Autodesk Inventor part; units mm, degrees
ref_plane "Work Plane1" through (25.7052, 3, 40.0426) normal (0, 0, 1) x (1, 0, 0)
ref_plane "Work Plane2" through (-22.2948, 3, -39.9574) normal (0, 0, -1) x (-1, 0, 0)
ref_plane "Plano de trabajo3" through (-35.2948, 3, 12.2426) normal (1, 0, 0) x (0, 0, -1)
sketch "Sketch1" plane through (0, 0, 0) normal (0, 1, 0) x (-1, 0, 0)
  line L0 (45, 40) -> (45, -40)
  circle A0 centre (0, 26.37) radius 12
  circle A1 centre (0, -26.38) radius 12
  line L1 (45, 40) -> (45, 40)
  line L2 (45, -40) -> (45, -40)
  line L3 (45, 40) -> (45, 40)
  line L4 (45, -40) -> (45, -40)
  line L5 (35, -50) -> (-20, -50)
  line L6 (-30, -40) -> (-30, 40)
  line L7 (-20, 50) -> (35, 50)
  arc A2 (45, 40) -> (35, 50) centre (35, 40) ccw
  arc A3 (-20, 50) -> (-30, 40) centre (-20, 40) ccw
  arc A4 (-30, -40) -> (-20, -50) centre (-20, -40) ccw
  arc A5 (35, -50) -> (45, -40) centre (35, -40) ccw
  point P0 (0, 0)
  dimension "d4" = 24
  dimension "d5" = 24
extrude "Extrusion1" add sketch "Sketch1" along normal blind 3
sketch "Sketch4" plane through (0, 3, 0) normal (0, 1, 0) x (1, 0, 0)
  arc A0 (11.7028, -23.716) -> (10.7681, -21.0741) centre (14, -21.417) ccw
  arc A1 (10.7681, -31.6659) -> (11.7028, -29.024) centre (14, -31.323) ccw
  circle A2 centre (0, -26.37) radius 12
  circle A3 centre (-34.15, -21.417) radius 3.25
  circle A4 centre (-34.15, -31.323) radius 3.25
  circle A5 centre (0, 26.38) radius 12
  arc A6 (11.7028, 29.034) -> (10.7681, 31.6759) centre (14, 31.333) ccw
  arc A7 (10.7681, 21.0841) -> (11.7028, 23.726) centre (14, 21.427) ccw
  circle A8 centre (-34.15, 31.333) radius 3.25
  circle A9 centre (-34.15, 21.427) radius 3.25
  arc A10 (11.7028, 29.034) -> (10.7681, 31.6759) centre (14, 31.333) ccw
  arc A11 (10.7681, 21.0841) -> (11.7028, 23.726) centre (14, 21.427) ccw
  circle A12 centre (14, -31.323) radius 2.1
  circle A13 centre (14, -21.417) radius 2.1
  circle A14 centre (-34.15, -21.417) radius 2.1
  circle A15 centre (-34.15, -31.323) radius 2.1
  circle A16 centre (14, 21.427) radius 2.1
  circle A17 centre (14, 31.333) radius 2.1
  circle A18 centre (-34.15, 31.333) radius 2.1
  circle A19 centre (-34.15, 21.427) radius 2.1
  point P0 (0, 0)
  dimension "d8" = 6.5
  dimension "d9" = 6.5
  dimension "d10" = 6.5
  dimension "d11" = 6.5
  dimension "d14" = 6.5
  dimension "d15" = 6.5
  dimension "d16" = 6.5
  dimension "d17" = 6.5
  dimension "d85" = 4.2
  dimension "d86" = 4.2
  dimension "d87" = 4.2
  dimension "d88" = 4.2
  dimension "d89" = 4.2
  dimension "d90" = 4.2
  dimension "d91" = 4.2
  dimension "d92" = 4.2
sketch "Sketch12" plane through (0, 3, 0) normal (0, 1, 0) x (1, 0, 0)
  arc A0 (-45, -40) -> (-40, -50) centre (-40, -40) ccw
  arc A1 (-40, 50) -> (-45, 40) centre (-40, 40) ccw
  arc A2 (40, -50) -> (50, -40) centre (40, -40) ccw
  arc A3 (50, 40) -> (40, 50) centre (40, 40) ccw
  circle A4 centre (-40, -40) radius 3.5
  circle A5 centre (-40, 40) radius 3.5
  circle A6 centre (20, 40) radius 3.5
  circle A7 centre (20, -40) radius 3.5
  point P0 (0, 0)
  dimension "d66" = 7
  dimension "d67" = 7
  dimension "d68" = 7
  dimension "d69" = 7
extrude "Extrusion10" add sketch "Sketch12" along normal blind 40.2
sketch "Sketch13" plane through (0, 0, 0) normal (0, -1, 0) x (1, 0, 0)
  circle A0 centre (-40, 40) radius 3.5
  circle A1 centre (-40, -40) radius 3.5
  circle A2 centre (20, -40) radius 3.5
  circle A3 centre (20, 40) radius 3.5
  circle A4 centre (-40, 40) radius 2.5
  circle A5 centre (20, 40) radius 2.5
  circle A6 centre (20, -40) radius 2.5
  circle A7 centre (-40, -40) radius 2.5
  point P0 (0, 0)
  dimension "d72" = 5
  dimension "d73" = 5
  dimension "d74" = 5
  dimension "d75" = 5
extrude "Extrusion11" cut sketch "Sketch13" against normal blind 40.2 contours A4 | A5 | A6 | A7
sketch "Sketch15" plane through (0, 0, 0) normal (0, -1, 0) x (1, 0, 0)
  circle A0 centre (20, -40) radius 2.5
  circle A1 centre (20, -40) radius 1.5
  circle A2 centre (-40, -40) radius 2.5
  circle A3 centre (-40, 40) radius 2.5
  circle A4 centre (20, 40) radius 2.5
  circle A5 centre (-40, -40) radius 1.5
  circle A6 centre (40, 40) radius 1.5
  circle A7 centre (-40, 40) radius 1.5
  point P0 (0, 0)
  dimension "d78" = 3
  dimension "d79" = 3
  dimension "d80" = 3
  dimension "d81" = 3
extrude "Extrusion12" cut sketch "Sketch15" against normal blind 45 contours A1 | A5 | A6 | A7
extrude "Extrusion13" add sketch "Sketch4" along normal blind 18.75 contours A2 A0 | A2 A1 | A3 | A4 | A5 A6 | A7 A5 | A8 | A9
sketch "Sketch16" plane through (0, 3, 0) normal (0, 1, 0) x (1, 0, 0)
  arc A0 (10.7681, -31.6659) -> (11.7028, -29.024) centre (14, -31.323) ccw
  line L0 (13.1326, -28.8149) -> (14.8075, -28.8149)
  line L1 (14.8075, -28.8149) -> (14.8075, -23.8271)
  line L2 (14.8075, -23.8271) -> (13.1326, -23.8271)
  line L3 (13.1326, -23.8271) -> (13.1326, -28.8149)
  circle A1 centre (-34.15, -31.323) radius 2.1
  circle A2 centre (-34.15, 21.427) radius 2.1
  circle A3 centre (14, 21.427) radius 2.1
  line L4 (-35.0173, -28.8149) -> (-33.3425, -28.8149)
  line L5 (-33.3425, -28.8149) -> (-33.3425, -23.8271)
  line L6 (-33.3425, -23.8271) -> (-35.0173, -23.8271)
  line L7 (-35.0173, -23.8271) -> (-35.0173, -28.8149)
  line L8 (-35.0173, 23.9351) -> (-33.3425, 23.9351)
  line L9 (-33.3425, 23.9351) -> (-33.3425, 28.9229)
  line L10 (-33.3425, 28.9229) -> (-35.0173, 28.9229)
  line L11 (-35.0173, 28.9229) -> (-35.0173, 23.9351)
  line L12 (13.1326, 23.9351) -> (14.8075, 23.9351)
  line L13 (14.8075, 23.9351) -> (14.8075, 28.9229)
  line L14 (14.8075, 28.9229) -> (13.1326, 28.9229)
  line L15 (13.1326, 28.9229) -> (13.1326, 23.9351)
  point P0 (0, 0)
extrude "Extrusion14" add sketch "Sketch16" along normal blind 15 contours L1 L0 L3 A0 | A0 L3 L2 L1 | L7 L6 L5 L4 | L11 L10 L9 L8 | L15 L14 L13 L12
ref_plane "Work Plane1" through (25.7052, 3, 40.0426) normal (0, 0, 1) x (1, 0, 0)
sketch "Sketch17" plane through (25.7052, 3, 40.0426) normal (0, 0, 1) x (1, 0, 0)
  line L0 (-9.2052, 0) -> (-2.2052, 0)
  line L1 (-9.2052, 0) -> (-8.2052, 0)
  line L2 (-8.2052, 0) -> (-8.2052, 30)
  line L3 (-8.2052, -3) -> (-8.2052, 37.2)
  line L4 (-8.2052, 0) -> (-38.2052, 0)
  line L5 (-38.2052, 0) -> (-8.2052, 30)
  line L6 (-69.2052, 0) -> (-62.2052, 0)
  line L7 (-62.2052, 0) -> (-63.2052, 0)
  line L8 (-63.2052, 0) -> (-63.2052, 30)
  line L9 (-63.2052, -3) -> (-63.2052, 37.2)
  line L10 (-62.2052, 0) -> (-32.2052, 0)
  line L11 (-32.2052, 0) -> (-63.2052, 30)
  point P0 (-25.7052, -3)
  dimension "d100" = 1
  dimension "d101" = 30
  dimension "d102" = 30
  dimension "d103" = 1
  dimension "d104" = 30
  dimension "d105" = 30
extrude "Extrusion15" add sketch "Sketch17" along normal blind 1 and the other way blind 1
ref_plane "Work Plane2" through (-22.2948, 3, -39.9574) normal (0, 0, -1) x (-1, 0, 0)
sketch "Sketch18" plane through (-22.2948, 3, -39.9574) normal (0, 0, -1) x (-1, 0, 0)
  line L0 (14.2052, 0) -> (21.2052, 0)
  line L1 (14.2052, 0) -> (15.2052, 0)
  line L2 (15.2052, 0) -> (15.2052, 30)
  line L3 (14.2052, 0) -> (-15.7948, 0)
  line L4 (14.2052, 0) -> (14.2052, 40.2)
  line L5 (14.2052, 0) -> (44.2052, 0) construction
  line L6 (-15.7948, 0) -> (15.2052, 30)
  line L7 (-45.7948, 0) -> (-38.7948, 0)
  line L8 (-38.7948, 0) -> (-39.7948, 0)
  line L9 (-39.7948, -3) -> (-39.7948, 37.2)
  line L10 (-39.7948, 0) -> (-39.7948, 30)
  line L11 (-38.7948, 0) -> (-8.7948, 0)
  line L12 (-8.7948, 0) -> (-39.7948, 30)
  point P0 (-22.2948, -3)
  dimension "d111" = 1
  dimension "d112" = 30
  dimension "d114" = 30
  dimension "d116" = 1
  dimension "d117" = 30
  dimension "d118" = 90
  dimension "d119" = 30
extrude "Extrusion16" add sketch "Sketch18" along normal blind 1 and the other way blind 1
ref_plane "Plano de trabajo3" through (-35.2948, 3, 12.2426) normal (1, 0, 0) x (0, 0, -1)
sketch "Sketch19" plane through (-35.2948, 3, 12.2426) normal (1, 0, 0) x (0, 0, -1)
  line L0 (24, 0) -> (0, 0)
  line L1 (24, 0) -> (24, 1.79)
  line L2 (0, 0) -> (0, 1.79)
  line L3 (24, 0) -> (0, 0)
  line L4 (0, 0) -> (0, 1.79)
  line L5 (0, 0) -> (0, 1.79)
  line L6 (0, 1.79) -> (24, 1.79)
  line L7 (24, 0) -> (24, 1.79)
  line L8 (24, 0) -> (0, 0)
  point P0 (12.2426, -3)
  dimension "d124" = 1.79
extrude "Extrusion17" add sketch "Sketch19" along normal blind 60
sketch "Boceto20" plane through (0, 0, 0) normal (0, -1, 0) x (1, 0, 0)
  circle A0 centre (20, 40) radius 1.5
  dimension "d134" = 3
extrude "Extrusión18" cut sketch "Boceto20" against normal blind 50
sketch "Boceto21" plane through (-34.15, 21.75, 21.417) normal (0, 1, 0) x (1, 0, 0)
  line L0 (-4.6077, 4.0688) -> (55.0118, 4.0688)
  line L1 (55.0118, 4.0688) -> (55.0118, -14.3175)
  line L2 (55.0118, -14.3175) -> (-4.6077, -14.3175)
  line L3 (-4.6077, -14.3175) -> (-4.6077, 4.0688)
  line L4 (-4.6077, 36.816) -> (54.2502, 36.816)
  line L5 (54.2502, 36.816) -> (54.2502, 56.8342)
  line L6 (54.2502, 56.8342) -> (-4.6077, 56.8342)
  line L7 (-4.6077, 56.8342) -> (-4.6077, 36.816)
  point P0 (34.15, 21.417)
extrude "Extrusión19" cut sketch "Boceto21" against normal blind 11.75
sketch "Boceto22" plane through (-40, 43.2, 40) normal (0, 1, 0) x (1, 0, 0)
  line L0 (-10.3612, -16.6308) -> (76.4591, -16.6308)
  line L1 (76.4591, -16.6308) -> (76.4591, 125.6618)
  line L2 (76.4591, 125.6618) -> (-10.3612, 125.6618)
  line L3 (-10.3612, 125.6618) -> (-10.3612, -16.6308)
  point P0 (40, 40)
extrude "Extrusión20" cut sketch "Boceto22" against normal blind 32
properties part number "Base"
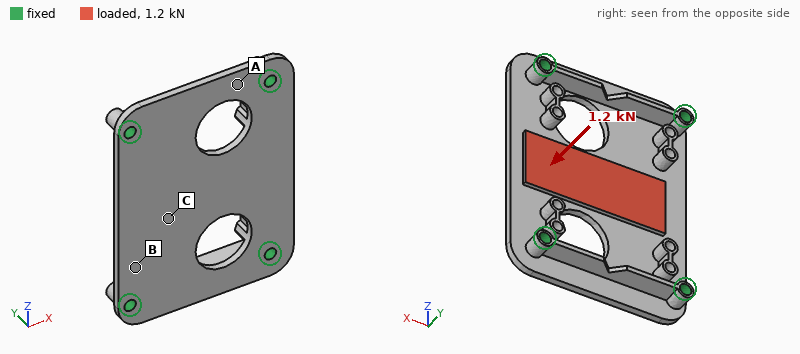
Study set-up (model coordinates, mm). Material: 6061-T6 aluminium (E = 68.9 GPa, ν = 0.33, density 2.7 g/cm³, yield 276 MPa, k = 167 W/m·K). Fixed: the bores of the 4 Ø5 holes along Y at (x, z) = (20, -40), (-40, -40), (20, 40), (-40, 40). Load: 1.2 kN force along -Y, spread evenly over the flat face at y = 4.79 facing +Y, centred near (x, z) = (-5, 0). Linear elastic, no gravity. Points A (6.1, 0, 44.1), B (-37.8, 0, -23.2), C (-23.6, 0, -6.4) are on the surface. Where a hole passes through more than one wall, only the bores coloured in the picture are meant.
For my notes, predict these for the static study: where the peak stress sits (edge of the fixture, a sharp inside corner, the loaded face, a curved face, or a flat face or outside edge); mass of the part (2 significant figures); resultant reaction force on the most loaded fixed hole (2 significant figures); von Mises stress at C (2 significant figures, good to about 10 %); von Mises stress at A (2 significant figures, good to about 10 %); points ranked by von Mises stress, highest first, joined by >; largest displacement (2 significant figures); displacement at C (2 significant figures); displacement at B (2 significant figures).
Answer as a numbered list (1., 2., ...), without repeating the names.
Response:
1. a flat face or outside edge
2. 68 g
3. 380 N
4. 34 MPa
5. 25 MPa
6. C > A > B
7. 0.23 mm
8. 0.20 mm
9. 0.084 mm
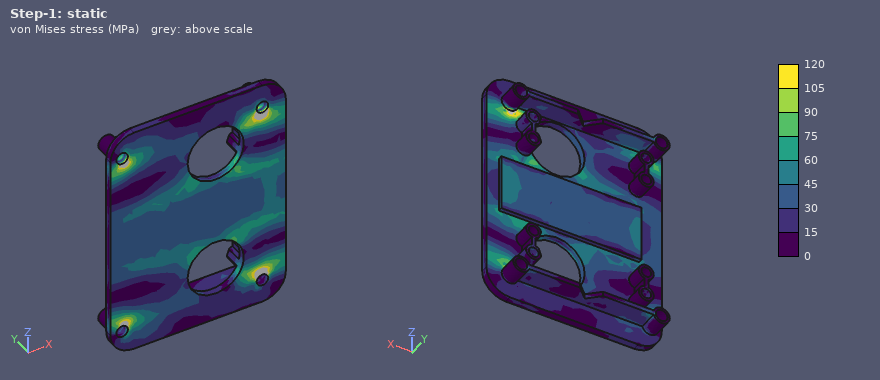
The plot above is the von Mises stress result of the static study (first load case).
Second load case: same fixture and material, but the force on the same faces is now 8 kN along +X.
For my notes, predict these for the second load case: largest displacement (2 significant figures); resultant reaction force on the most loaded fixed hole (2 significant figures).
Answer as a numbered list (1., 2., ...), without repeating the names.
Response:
1. 0.22 mm
2. 3.0 kN
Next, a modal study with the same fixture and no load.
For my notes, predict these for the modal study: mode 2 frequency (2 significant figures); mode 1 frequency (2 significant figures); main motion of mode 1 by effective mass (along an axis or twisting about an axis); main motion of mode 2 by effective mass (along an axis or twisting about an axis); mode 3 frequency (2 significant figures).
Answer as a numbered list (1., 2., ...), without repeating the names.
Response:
1. 3100 Hz
2. 2200 Hz
3. along Y
4. twisting about Z
5. 5900 Hz
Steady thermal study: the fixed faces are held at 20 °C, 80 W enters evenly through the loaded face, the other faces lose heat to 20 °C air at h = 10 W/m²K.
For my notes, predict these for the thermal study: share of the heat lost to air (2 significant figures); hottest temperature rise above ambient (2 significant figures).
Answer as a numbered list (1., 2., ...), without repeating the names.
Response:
1. 4.7 %
2. 54 K
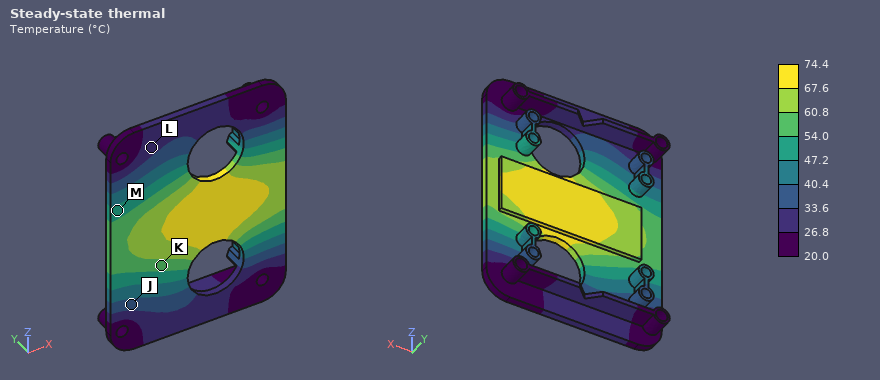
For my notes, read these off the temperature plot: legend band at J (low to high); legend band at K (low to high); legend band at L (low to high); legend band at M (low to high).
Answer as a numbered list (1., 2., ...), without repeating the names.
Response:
1. 33.6 to 40.4 °C
2. 54.0 to 60.8 °C
3. 26.8 to 33.6 °C
4. 47.2 to 54.0 °C
